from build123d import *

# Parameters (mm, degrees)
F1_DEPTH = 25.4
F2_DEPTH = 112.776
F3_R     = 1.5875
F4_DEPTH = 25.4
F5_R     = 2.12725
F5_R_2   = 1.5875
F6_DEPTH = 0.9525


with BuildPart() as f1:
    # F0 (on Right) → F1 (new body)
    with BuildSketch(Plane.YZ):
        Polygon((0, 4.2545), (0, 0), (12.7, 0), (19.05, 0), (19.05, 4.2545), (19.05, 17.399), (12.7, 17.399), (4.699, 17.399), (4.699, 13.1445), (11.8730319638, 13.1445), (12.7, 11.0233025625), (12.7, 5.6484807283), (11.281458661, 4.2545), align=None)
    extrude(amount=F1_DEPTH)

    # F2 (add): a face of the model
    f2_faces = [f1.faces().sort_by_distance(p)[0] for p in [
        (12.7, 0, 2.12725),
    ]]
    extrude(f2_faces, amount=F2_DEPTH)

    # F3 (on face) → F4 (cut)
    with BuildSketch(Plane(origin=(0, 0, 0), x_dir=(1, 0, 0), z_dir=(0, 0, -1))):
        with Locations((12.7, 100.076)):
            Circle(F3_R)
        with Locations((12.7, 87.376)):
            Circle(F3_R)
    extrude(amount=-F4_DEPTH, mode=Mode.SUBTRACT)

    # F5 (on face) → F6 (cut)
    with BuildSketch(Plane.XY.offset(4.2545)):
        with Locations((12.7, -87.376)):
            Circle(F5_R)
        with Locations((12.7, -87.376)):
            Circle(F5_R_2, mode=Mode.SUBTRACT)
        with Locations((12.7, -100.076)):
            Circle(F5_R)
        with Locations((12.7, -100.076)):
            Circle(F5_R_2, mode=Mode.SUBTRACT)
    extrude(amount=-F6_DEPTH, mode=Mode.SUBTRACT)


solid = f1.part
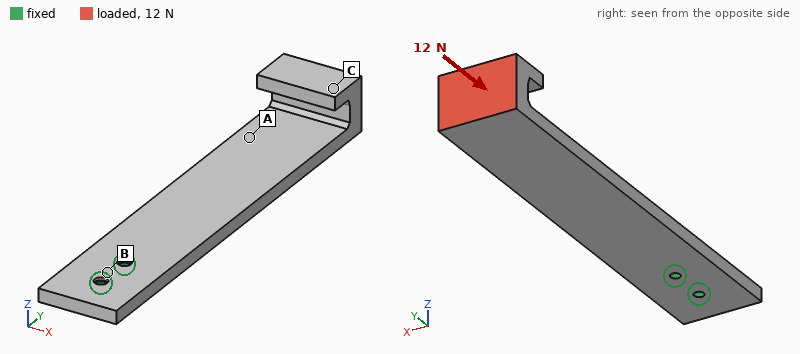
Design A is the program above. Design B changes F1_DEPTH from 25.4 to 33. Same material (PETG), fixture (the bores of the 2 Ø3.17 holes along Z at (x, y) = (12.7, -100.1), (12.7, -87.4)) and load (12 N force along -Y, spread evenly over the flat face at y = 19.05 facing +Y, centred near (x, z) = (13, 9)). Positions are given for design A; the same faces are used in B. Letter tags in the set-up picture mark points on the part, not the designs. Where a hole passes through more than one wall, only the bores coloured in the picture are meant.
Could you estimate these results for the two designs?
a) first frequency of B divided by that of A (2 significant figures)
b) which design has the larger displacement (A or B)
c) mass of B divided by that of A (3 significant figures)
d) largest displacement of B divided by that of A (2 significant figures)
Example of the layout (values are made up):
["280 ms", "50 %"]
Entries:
["0.99", "A", "1.30", "0.78"]
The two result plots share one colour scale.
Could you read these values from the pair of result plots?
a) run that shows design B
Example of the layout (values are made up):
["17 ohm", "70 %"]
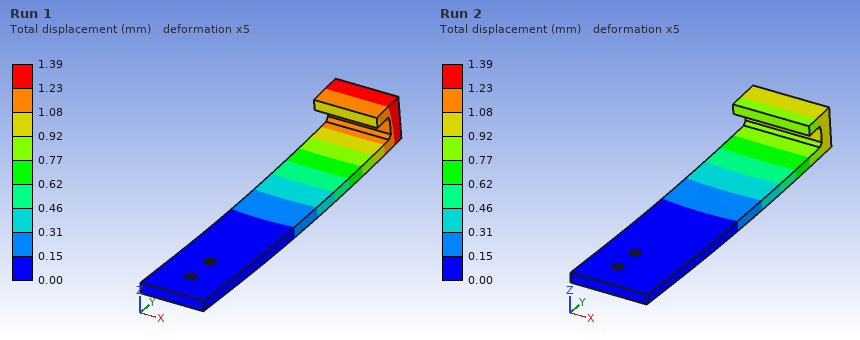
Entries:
["Run 2"]
